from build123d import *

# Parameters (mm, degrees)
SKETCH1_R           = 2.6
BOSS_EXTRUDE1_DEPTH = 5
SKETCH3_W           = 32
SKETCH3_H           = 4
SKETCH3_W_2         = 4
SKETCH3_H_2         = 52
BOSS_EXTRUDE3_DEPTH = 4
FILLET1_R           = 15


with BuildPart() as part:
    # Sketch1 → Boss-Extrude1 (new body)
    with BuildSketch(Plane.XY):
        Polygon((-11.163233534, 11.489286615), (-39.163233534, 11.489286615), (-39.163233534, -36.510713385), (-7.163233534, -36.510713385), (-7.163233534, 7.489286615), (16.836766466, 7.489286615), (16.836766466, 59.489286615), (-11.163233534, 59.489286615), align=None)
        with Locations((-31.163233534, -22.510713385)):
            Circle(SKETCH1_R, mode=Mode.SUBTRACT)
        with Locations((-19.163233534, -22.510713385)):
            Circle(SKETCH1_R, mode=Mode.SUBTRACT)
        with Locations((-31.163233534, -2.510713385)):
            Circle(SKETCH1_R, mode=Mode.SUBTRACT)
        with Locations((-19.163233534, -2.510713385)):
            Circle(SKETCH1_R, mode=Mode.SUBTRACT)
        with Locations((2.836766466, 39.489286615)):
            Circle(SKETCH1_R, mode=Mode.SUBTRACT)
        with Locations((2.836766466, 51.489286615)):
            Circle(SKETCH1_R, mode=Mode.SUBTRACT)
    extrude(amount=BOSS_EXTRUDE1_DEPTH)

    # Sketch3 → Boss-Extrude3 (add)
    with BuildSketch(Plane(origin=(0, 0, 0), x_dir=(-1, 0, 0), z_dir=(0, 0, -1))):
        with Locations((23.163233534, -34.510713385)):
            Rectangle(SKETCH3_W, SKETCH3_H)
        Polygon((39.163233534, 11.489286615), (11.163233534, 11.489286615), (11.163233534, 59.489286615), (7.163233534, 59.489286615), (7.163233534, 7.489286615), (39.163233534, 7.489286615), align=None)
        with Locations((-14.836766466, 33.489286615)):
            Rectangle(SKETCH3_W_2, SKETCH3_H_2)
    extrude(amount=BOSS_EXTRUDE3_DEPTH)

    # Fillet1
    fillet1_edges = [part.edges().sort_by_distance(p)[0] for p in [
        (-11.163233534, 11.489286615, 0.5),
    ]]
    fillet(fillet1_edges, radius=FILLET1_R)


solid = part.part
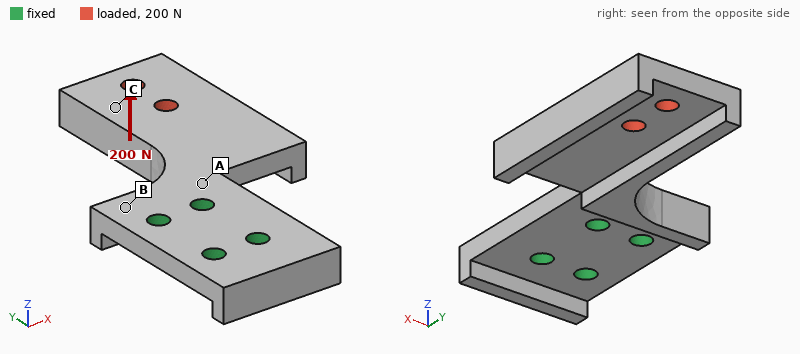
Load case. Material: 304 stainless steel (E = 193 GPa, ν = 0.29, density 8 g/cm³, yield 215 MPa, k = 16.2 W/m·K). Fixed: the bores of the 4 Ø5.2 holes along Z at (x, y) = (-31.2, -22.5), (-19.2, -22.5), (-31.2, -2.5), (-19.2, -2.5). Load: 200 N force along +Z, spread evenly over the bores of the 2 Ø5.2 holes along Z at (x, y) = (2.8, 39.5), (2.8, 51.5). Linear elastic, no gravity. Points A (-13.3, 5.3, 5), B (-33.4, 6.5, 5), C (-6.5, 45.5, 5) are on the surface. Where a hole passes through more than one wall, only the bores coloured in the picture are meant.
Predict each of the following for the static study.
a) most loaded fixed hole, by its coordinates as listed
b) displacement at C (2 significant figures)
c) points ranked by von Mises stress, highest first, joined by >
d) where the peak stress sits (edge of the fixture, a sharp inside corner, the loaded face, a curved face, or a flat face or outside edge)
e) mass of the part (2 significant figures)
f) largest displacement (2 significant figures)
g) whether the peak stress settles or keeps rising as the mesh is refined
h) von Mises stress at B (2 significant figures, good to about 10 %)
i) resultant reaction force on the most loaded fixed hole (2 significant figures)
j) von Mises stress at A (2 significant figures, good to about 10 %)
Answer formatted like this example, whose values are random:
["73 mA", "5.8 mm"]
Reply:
["(-19.2, -2.5)", "0.13 mm", "A > B > C", "edge of the fixture", "140 g", "0.22 mm", "keeps rising", "36 MPa", "450 N", "85 MPa"]
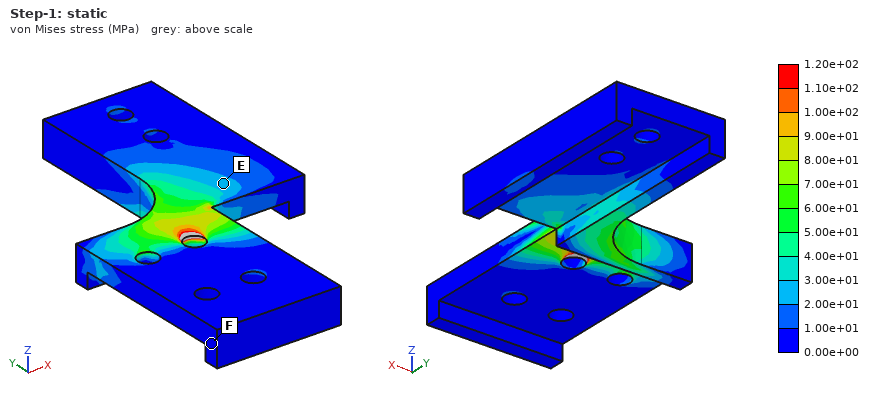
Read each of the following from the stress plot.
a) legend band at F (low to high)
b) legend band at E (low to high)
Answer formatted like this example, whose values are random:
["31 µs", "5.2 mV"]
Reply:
["0.00e+00 to 1.00e+01 MPa", "2.00e+01 to 3.00e+01 MPa"]
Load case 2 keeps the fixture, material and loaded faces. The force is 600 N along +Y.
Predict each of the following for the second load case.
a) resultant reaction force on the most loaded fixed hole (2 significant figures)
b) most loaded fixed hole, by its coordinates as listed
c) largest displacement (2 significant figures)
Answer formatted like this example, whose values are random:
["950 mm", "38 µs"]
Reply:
["770 N", "(-19.2, -2.5)", "44 µm"]
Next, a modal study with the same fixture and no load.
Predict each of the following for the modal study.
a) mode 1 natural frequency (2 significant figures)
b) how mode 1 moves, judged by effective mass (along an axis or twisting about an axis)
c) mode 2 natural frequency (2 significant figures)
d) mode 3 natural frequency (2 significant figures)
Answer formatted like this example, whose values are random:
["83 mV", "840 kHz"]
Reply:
["870 Hz", "along Z", "2000 Hz", "2800 Hz"]
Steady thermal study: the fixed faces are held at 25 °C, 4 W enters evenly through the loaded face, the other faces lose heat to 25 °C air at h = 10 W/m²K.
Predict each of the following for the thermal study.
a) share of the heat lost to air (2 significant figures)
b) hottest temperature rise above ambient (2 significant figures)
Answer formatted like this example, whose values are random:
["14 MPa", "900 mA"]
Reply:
["52 %", "63 K"]
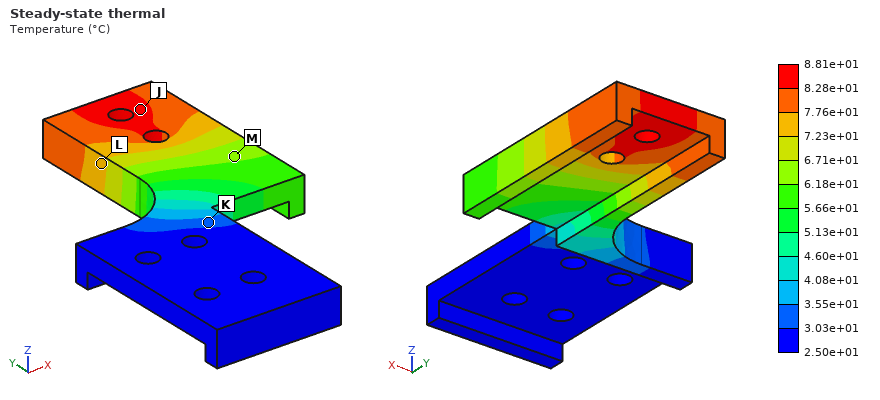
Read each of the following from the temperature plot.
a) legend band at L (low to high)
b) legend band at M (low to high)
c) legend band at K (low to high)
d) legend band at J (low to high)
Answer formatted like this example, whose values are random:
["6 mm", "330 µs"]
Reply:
["7.23e+01 to 7.76e+01 °C", "6.18e+01 to 6.71e+01 °C", "3.03e+01 to 3.55e+01 °C", "8.28e+01 to 8.81e+01 °C"]
